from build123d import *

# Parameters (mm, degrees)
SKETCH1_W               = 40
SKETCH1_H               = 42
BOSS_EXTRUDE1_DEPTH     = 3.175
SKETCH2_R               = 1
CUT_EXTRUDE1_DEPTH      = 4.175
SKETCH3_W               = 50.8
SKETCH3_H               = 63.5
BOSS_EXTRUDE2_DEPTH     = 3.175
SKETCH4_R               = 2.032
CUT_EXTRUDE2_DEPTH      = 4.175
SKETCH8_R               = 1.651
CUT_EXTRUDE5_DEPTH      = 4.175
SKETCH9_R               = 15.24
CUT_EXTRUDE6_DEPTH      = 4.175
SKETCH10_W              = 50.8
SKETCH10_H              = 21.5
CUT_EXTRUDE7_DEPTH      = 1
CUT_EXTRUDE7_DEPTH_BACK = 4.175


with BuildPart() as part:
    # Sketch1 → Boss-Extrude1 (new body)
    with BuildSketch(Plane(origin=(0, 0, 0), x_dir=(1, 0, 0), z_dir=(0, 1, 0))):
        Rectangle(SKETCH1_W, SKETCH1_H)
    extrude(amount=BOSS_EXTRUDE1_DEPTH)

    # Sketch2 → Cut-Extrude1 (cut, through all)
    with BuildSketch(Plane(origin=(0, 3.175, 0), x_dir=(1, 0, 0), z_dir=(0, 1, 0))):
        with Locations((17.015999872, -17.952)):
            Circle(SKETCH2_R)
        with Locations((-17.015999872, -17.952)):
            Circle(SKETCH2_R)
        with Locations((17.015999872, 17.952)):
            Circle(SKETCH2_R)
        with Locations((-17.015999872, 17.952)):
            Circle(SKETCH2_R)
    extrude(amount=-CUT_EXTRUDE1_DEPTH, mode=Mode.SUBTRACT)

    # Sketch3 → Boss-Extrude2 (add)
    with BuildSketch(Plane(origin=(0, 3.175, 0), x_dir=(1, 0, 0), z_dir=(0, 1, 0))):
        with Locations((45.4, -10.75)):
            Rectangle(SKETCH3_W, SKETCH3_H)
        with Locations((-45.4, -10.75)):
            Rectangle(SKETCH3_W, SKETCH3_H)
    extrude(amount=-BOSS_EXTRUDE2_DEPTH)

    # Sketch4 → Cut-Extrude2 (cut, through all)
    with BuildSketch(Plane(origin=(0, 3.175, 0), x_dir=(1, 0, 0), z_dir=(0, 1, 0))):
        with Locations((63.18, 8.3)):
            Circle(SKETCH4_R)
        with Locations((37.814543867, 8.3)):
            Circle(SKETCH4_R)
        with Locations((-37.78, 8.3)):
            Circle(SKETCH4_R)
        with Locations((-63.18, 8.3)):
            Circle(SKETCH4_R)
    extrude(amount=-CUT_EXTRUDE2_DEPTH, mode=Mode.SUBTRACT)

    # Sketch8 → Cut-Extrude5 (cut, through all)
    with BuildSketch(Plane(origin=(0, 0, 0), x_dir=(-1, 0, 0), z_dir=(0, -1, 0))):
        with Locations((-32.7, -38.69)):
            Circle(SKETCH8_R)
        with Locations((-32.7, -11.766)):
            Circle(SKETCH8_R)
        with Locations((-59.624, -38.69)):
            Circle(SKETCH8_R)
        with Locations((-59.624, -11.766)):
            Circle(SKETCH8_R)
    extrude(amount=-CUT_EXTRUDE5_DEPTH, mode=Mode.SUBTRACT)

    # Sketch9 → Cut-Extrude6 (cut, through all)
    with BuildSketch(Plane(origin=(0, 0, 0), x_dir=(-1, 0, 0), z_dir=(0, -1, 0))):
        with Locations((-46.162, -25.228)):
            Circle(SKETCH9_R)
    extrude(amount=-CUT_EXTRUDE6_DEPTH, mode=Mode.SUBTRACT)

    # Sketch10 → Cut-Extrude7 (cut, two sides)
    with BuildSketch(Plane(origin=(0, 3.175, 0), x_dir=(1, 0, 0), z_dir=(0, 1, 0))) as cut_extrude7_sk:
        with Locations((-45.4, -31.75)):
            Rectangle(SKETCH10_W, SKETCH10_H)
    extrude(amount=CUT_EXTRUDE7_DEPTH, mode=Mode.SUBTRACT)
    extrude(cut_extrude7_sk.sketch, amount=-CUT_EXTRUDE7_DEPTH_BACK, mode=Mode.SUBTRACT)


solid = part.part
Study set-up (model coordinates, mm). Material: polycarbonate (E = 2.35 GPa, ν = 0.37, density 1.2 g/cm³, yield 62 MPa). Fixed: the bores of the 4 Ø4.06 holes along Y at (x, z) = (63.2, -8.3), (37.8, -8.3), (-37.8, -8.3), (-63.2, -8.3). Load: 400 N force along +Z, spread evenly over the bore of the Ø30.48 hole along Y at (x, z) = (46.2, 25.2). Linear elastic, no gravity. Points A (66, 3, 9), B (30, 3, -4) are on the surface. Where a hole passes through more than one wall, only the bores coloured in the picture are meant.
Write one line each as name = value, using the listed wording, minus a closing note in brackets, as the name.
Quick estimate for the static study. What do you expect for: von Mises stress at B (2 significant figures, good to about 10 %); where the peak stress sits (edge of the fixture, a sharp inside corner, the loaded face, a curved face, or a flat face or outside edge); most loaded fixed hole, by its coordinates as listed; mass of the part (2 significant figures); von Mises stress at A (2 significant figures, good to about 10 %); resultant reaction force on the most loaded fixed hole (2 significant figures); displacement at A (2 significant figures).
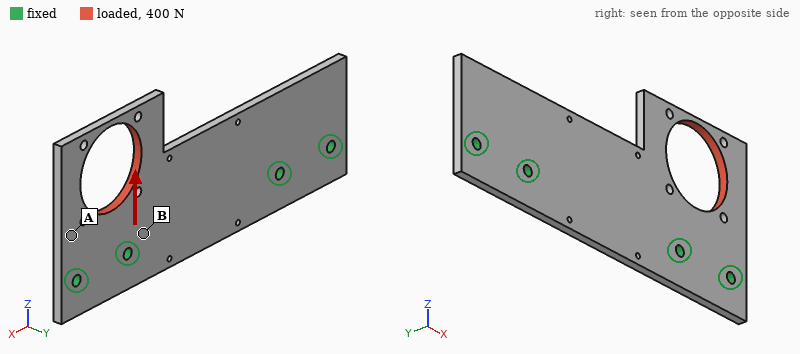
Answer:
von Mises stress at B = 2.1 MPa
where the peak stress sits = a flat face or outside edge
most loaded fixed hole, by its coordinates as listed = (63.2, -8.3)
mass of the part = 24 g
von Mises stress at A = 5.2 MPa
resultant reaction force on the most loaded fixed hole = 210 N
displacement at A = 0.049 mm
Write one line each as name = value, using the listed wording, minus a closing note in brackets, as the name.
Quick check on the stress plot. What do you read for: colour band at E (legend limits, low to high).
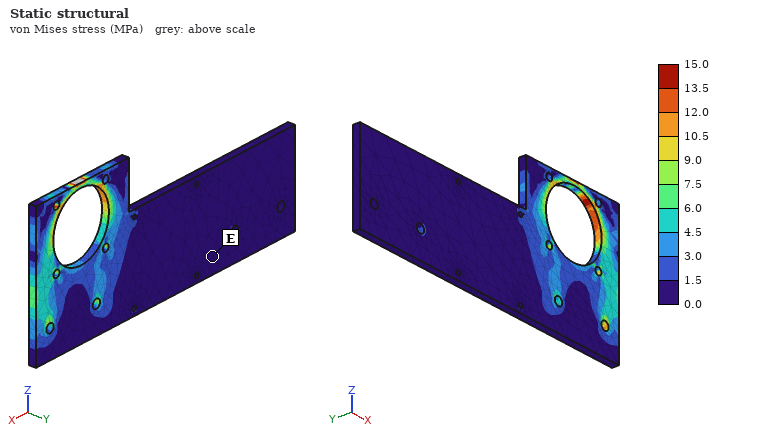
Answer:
colour band at E = 0.0 to 1.5 MPa
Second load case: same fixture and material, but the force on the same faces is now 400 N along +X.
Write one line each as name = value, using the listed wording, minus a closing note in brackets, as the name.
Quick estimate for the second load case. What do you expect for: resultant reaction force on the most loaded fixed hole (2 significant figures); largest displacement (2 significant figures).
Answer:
resultant reaction force on the most loaded fixed hole = 240 N
largest displacement = 0.72 mm
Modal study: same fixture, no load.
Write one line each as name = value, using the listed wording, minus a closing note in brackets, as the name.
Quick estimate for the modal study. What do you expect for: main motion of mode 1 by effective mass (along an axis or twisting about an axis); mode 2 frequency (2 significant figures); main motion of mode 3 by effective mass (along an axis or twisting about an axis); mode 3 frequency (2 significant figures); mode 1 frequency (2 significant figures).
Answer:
main motion of mode 1 by effective mass = along Y
mode 2 frequency = 520 Hz
main motion of mode 3 by effective mass = along Y
mode 3 frequency = 770 Hz
mode 1 frequency = 340 Hz
